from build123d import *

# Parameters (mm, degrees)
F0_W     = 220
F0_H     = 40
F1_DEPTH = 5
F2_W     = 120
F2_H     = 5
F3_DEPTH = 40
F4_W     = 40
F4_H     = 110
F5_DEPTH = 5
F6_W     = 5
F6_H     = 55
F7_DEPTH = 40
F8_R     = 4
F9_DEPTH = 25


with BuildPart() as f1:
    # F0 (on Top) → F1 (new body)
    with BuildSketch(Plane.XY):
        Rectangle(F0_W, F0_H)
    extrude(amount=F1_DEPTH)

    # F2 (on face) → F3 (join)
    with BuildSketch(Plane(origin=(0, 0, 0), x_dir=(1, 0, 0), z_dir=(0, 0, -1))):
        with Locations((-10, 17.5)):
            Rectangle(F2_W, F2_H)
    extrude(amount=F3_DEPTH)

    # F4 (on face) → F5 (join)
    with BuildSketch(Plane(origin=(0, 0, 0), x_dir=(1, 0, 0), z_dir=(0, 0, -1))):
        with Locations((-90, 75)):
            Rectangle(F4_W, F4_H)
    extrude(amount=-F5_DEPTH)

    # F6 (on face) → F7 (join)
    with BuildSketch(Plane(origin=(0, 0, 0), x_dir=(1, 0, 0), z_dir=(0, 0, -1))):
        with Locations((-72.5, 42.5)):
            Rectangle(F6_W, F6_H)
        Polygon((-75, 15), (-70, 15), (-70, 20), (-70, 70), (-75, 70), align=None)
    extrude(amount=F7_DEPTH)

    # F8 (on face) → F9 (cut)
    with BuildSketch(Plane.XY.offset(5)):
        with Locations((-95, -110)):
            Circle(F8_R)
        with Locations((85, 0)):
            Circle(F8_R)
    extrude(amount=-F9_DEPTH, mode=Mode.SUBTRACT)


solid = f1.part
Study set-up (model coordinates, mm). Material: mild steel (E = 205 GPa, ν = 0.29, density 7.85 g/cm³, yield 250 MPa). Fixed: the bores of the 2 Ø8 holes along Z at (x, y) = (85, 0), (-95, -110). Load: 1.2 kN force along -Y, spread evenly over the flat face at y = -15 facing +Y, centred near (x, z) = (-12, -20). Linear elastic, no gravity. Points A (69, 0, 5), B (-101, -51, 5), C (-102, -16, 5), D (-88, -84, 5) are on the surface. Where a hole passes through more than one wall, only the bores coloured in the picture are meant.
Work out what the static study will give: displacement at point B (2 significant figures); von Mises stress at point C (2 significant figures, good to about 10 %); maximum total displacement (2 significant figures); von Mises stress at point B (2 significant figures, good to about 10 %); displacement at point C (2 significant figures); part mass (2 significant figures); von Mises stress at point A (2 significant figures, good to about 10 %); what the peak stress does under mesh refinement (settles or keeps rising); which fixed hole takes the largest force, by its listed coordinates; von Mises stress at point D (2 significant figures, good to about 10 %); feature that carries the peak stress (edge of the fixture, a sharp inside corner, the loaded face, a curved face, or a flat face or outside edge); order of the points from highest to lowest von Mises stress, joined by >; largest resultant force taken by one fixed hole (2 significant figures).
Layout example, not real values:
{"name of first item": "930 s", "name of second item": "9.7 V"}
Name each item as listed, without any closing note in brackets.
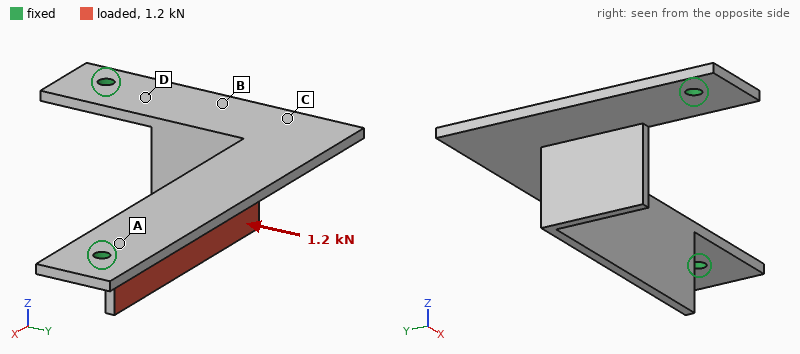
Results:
{"displacement at point B": "0.16 mm", "von Mises stress at point C": "8.3 MPa", "maximum total displacement": "0.53 mm", "von Mises stress at point B": "16 MPa", "displacement at point C": "0.33 mm", "part mass": "790 g", "von Mises stress at point A": "69 MPa", "what the peak stress does under mesh refinement": "keeps rising", "which fixed hole takes the largest force, by its listed coordinates": "(-95, -110)", "von Mises stress at point D": "55 MPa", "feature that carries the peak stress": "edge of the fixture", "order of the points from highest to lowest von Mises stress, joined by >": "A > D > B > C", "largest resultant force taken by one fixed hole": "790 N"}
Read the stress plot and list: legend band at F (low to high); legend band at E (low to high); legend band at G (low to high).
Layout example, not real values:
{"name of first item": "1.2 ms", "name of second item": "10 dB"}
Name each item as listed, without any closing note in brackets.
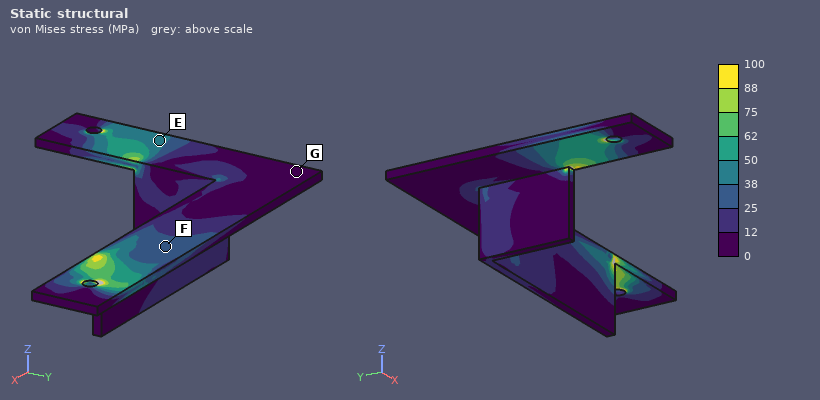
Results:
{"legend band at F": "25 to 38 MPa", "legend band at E": "38 to 50 MPa", "legend band at G": "0 to 12 MPa"}
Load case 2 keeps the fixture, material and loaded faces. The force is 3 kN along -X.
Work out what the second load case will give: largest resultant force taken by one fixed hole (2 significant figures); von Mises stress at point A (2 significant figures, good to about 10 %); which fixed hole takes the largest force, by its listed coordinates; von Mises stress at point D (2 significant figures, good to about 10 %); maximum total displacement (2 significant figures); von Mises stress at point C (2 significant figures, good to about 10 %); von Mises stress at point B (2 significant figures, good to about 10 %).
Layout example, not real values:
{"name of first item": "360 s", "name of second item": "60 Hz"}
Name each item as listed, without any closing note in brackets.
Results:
{"largest resultant force taken by one fixed hole": "2.9 kN", "von Mises stress at point A": "83 MPa", "which fixed hole takes the largest force, by its listed coordinates": "(85, 0)", "von Mises stress at point D": "81 MPa", "maximum total displacement": "0.89 mm", "von Mises stress at point C": "25 MPa", "von Mises stress at point B": "30 MPa"}
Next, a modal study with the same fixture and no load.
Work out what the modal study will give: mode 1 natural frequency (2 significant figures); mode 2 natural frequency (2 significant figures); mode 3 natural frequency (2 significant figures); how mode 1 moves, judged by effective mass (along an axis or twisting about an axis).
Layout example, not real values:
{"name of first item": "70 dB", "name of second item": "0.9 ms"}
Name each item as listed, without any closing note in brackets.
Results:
{"mode 1 natural frequency": "250 Hz", "mode 2 natural frequency": "1100 Hz", "mode 3 natural frequency": "1300 Hz", "how mode 1 moves, judged by effective mass": "along Z"}
